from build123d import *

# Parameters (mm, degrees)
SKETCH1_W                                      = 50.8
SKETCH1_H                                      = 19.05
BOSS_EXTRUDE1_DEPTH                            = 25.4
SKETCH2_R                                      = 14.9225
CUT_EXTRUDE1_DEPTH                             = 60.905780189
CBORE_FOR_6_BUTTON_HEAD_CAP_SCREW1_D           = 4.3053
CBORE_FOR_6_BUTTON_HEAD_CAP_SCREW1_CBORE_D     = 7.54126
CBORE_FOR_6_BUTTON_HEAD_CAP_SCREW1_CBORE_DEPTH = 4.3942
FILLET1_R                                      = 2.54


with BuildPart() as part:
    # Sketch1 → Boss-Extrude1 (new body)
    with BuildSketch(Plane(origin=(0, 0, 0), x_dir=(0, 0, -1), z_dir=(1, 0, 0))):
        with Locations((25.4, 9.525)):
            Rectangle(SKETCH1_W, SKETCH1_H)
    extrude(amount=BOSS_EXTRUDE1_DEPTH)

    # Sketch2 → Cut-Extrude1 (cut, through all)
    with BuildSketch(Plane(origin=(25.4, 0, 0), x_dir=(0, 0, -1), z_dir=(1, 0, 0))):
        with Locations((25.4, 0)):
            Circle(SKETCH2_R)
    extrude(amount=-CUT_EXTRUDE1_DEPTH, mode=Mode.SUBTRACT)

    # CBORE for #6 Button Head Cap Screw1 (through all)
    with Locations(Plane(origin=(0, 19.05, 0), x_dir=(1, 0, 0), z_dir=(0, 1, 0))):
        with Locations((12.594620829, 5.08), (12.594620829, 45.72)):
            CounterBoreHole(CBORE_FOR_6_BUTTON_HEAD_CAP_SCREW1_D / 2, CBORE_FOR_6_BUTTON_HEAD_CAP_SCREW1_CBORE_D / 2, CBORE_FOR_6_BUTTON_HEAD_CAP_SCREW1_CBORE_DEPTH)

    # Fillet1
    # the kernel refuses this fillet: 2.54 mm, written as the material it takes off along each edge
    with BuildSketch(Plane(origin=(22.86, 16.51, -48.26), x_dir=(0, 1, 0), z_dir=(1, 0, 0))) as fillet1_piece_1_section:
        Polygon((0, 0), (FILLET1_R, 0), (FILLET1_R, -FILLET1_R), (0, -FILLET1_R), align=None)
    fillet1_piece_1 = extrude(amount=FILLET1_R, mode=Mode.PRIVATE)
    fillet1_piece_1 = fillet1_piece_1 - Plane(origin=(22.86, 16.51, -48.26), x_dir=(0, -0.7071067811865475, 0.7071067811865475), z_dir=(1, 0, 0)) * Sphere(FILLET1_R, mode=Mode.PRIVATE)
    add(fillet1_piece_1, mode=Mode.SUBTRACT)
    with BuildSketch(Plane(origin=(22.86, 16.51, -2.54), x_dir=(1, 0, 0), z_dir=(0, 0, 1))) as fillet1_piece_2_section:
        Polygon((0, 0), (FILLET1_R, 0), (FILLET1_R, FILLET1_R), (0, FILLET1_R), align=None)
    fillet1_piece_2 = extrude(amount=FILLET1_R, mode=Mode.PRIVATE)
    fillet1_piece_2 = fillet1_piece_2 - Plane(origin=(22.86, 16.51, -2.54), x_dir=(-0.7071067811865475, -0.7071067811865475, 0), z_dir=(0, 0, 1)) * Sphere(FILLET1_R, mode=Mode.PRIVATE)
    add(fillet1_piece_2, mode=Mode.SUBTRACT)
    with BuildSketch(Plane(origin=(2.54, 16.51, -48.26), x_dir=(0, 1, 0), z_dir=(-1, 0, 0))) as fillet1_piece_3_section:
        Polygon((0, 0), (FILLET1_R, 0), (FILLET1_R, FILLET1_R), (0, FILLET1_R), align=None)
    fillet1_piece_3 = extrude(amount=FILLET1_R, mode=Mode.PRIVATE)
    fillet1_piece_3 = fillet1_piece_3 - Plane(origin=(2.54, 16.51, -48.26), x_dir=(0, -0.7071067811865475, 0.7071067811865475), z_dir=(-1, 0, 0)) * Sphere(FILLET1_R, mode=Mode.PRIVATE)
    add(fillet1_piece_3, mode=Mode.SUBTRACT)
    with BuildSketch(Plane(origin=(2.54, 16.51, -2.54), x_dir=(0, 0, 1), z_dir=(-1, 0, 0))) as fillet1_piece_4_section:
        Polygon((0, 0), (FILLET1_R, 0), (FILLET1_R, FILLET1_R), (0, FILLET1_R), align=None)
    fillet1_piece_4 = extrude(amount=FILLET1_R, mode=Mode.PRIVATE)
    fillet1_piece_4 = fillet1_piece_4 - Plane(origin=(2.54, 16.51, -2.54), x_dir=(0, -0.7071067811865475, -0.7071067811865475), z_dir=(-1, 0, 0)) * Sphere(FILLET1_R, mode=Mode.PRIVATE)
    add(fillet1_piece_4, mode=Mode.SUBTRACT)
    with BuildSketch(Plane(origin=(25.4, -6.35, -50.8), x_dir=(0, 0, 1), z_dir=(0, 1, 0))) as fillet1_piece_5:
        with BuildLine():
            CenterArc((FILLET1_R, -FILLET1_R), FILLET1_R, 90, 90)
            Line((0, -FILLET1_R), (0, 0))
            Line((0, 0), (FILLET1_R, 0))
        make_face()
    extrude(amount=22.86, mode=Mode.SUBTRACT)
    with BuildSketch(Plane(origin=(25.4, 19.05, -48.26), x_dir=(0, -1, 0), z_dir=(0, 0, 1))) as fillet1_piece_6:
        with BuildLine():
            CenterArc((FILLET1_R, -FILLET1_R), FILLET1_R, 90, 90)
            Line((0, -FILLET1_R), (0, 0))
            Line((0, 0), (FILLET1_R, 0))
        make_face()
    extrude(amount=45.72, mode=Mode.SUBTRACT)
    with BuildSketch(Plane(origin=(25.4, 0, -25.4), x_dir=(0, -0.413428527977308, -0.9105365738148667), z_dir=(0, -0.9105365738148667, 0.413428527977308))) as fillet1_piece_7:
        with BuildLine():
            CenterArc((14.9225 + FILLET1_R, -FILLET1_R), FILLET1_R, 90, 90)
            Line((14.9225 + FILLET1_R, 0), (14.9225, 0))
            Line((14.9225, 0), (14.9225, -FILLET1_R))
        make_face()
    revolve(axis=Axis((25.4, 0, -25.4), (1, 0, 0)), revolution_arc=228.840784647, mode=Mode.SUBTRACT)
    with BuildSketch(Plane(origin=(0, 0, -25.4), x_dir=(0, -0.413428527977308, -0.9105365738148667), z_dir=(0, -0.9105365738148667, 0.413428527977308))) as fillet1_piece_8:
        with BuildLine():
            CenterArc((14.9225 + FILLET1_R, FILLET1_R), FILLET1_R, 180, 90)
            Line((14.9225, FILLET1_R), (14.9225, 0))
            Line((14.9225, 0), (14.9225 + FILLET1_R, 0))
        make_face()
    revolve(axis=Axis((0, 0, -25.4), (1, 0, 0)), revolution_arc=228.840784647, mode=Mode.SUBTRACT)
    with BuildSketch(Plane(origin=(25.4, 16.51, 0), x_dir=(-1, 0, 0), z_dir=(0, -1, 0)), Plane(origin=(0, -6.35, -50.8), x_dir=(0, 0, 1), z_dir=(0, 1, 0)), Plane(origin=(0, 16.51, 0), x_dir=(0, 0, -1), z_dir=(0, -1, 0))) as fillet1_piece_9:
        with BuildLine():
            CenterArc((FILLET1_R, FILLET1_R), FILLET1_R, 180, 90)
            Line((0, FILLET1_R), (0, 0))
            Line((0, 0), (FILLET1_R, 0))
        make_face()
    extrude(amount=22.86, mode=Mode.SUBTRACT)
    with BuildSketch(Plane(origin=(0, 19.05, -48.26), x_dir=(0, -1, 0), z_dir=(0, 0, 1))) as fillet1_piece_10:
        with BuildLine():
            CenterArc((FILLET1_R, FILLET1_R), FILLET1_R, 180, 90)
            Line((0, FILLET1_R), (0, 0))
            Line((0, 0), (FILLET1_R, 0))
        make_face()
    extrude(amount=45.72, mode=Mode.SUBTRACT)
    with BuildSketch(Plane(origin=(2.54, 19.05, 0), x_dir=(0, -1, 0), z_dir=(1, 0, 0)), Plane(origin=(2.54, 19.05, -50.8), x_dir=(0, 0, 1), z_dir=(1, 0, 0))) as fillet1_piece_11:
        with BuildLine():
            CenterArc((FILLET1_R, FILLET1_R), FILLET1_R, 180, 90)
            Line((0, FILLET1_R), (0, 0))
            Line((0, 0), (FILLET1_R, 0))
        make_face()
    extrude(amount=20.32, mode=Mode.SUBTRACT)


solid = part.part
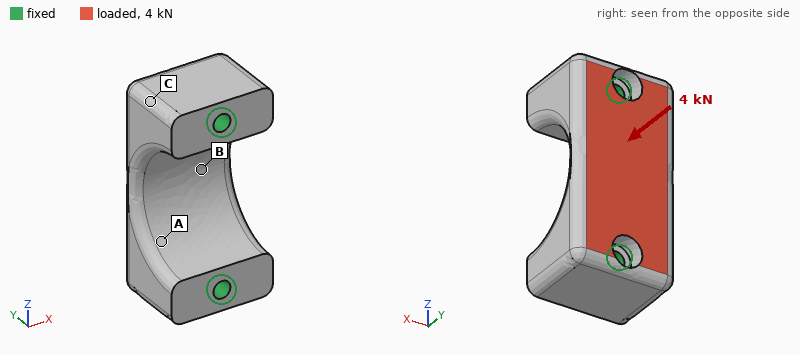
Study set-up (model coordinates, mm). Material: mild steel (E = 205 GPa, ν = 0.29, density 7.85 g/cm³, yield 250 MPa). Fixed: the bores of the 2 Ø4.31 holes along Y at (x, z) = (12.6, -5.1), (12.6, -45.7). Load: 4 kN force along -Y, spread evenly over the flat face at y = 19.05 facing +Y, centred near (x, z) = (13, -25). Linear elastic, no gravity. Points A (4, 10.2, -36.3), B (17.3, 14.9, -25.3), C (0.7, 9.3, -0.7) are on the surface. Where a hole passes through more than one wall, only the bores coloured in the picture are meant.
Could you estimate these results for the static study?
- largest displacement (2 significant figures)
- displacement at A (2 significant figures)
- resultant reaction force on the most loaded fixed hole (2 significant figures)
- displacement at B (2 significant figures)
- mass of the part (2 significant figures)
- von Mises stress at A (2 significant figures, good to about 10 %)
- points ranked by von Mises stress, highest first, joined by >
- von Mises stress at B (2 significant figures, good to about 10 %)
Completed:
3.5 µm
1.5 µm
2.3 kN
3.4 µm
110 g
18 MPa
A > B > C
8.8 MPa
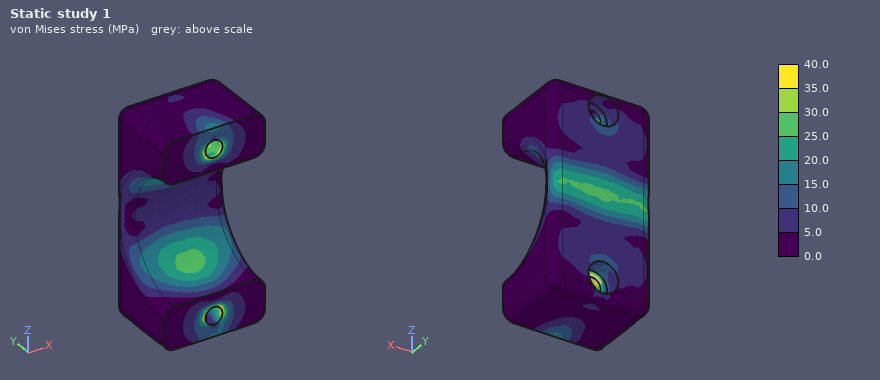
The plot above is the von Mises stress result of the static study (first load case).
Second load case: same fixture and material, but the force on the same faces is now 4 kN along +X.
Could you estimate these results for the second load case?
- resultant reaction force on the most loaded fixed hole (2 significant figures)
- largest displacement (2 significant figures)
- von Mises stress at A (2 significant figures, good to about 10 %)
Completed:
2.0 kN
6.7 µm
14 MPa
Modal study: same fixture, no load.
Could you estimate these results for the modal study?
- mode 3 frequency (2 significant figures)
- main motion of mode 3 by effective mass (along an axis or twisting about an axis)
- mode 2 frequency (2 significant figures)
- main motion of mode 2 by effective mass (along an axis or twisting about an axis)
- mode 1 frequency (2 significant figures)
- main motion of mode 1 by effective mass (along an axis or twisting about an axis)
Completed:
32 kHz
along Z
29 kHz
along Y
22 kHz
along X
